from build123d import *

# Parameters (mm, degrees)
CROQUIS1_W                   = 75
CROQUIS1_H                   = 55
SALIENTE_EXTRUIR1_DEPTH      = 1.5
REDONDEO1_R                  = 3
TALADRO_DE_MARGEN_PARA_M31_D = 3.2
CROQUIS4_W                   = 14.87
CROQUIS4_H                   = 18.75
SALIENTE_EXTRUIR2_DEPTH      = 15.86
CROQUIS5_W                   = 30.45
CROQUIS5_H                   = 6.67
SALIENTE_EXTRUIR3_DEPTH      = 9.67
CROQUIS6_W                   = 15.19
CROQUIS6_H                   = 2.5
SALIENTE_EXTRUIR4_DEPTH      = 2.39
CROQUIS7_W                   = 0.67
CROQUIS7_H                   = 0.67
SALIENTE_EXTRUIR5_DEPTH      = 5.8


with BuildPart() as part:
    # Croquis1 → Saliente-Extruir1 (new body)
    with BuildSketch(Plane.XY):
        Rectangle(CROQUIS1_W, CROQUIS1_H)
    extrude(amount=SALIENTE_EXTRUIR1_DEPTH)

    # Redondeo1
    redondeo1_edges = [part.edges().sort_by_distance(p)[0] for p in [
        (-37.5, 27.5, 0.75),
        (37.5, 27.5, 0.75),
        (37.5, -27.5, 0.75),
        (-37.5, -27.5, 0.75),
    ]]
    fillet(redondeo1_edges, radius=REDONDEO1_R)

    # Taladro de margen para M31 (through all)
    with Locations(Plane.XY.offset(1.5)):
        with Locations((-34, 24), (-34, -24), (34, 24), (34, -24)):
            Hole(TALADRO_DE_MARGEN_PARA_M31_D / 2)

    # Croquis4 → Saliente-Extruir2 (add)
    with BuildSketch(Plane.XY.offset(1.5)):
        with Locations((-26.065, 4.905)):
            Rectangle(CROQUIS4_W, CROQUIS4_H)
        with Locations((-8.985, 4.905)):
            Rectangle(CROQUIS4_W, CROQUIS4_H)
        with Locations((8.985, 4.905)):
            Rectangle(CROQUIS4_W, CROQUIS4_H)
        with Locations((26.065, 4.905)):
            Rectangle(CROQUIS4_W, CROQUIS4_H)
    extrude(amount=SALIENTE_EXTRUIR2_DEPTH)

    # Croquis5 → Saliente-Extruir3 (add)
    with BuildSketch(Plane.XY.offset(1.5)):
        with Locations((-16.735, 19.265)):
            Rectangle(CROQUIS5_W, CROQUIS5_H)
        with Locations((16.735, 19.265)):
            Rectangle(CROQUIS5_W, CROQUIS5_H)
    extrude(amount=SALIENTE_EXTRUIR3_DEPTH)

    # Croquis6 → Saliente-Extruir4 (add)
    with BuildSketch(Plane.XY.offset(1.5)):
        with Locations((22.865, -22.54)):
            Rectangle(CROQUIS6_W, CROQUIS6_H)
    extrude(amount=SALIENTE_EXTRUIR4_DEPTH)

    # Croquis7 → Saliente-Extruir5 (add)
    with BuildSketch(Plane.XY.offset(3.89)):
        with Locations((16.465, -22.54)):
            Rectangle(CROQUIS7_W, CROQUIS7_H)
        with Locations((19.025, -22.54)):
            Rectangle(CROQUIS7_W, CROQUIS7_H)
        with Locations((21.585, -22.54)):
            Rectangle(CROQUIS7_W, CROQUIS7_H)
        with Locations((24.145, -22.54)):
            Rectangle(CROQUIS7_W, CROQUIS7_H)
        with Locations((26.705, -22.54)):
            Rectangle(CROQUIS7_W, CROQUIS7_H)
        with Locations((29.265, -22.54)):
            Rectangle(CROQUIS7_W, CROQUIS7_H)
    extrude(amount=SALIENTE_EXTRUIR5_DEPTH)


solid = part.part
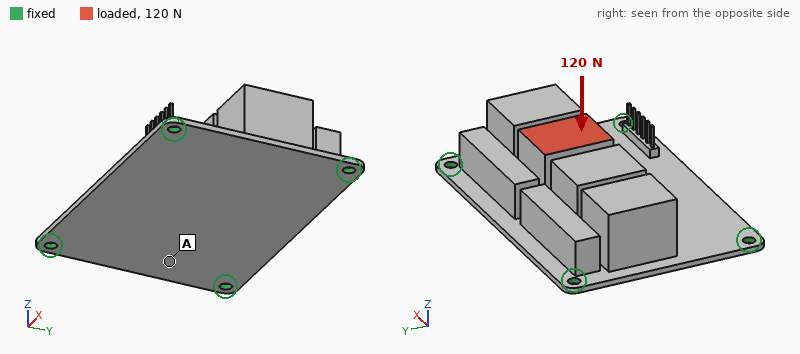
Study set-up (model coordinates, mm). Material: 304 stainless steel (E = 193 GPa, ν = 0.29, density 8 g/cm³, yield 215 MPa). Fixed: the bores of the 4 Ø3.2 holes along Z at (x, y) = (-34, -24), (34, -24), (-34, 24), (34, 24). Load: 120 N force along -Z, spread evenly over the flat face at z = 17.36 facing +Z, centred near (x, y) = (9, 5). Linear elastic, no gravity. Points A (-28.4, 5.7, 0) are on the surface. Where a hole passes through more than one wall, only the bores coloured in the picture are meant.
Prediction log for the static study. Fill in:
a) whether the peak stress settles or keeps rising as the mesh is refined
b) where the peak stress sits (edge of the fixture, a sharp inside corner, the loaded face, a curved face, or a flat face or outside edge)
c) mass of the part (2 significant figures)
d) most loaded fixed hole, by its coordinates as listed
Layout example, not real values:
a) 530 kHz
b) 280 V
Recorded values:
a) keeps rising
b) edge of the fixture
c) 220 g
d) (34, 24)
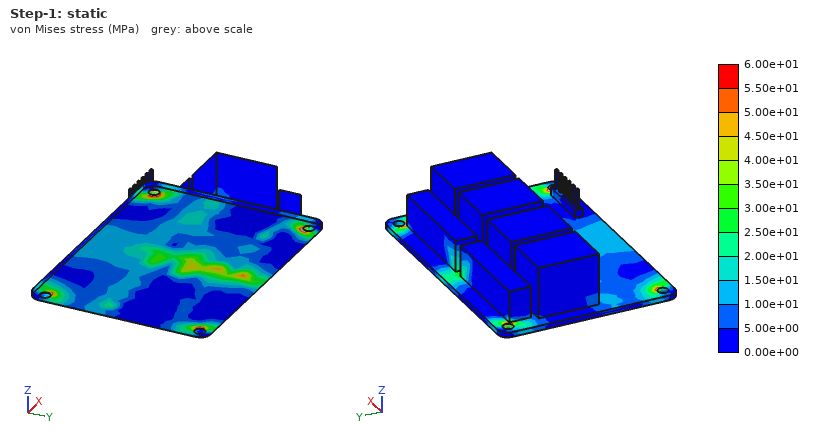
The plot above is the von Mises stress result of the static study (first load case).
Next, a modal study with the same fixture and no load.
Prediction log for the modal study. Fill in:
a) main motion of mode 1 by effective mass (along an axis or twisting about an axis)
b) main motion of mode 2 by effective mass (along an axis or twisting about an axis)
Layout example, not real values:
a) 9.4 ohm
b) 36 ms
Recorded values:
a) along Z
b) along Y
